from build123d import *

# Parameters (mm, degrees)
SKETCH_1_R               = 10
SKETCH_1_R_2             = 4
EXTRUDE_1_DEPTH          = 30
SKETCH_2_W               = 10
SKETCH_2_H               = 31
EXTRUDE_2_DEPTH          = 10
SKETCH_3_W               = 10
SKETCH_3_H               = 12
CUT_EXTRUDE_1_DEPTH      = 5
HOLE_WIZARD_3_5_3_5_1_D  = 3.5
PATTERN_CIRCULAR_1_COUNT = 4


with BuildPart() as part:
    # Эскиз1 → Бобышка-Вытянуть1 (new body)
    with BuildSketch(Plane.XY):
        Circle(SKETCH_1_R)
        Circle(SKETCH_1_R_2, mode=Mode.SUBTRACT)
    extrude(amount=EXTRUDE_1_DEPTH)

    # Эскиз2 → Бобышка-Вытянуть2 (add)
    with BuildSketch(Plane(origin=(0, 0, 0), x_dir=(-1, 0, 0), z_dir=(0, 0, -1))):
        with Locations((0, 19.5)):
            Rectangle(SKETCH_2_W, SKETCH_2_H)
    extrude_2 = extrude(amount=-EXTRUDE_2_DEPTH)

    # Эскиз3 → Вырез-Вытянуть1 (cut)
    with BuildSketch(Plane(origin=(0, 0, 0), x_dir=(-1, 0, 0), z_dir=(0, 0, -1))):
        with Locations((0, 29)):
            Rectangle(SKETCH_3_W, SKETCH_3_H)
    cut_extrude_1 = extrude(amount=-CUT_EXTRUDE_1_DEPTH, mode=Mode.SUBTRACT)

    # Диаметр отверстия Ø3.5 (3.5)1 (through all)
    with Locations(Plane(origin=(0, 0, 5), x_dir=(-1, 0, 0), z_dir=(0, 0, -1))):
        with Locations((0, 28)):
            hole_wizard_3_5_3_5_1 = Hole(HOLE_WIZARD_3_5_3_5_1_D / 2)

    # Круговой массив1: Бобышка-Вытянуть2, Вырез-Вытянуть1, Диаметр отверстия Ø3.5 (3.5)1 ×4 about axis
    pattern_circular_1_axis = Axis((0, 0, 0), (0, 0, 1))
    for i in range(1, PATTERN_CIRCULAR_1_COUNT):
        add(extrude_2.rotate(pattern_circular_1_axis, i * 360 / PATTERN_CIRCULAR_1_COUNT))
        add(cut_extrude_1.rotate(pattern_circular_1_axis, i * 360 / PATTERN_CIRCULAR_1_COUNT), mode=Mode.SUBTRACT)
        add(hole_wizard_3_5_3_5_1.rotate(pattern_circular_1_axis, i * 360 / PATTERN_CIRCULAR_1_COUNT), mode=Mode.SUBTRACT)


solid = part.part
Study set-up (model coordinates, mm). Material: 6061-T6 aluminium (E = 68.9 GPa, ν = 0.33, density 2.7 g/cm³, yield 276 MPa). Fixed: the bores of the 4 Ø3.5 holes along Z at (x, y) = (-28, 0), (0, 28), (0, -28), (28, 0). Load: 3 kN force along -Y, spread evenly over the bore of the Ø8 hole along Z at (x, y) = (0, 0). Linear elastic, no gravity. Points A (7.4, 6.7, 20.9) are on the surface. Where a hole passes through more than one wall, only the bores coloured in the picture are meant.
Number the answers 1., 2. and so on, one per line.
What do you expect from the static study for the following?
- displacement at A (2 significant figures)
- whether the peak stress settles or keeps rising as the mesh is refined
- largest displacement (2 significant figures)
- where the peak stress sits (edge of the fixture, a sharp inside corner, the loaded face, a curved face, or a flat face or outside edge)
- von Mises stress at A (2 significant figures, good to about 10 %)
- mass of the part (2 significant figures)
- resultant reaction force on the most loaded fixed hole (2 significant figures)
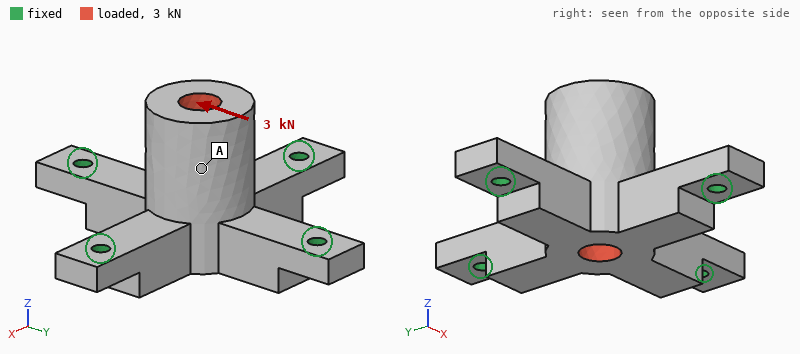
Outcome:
1. 31 µm
2. keeps rising
3. 46 µm
4. edge of the fixture
5. 6.9 MPa
6. 42 g
7. 1.4 kN
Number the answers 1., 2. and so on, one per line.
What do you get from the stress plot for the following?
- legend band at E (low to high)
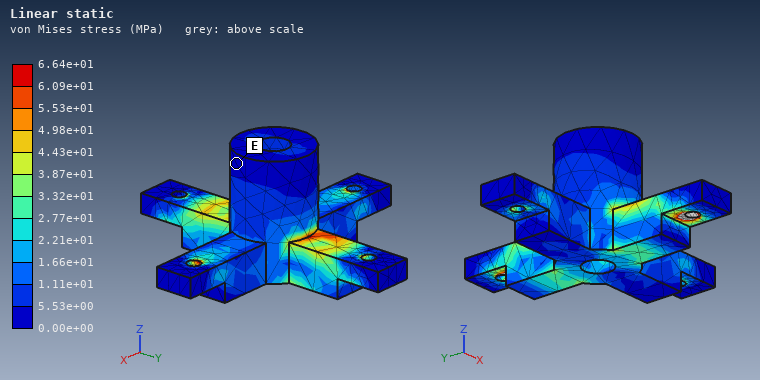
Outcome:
1. 0.00e+00 to 5.53e+00 MPa
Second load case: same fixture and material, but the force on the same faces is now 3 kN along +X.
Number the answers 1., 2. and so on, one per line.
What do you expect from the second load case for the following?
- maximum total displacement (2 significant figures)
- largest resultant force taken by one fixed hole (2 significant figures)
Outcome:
1. 47 µm
2. 1.4 kN
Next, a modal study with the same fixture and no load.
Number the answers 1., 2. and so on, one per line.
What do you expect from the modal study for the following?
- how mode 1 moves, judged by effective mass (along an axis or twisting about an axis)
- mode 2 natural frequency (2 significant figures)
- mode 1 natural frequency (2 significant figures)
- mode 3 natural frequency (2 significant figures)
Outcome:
1. along Z
2. 10 kHz
3. 9600 Hz
4. 10 kHz
